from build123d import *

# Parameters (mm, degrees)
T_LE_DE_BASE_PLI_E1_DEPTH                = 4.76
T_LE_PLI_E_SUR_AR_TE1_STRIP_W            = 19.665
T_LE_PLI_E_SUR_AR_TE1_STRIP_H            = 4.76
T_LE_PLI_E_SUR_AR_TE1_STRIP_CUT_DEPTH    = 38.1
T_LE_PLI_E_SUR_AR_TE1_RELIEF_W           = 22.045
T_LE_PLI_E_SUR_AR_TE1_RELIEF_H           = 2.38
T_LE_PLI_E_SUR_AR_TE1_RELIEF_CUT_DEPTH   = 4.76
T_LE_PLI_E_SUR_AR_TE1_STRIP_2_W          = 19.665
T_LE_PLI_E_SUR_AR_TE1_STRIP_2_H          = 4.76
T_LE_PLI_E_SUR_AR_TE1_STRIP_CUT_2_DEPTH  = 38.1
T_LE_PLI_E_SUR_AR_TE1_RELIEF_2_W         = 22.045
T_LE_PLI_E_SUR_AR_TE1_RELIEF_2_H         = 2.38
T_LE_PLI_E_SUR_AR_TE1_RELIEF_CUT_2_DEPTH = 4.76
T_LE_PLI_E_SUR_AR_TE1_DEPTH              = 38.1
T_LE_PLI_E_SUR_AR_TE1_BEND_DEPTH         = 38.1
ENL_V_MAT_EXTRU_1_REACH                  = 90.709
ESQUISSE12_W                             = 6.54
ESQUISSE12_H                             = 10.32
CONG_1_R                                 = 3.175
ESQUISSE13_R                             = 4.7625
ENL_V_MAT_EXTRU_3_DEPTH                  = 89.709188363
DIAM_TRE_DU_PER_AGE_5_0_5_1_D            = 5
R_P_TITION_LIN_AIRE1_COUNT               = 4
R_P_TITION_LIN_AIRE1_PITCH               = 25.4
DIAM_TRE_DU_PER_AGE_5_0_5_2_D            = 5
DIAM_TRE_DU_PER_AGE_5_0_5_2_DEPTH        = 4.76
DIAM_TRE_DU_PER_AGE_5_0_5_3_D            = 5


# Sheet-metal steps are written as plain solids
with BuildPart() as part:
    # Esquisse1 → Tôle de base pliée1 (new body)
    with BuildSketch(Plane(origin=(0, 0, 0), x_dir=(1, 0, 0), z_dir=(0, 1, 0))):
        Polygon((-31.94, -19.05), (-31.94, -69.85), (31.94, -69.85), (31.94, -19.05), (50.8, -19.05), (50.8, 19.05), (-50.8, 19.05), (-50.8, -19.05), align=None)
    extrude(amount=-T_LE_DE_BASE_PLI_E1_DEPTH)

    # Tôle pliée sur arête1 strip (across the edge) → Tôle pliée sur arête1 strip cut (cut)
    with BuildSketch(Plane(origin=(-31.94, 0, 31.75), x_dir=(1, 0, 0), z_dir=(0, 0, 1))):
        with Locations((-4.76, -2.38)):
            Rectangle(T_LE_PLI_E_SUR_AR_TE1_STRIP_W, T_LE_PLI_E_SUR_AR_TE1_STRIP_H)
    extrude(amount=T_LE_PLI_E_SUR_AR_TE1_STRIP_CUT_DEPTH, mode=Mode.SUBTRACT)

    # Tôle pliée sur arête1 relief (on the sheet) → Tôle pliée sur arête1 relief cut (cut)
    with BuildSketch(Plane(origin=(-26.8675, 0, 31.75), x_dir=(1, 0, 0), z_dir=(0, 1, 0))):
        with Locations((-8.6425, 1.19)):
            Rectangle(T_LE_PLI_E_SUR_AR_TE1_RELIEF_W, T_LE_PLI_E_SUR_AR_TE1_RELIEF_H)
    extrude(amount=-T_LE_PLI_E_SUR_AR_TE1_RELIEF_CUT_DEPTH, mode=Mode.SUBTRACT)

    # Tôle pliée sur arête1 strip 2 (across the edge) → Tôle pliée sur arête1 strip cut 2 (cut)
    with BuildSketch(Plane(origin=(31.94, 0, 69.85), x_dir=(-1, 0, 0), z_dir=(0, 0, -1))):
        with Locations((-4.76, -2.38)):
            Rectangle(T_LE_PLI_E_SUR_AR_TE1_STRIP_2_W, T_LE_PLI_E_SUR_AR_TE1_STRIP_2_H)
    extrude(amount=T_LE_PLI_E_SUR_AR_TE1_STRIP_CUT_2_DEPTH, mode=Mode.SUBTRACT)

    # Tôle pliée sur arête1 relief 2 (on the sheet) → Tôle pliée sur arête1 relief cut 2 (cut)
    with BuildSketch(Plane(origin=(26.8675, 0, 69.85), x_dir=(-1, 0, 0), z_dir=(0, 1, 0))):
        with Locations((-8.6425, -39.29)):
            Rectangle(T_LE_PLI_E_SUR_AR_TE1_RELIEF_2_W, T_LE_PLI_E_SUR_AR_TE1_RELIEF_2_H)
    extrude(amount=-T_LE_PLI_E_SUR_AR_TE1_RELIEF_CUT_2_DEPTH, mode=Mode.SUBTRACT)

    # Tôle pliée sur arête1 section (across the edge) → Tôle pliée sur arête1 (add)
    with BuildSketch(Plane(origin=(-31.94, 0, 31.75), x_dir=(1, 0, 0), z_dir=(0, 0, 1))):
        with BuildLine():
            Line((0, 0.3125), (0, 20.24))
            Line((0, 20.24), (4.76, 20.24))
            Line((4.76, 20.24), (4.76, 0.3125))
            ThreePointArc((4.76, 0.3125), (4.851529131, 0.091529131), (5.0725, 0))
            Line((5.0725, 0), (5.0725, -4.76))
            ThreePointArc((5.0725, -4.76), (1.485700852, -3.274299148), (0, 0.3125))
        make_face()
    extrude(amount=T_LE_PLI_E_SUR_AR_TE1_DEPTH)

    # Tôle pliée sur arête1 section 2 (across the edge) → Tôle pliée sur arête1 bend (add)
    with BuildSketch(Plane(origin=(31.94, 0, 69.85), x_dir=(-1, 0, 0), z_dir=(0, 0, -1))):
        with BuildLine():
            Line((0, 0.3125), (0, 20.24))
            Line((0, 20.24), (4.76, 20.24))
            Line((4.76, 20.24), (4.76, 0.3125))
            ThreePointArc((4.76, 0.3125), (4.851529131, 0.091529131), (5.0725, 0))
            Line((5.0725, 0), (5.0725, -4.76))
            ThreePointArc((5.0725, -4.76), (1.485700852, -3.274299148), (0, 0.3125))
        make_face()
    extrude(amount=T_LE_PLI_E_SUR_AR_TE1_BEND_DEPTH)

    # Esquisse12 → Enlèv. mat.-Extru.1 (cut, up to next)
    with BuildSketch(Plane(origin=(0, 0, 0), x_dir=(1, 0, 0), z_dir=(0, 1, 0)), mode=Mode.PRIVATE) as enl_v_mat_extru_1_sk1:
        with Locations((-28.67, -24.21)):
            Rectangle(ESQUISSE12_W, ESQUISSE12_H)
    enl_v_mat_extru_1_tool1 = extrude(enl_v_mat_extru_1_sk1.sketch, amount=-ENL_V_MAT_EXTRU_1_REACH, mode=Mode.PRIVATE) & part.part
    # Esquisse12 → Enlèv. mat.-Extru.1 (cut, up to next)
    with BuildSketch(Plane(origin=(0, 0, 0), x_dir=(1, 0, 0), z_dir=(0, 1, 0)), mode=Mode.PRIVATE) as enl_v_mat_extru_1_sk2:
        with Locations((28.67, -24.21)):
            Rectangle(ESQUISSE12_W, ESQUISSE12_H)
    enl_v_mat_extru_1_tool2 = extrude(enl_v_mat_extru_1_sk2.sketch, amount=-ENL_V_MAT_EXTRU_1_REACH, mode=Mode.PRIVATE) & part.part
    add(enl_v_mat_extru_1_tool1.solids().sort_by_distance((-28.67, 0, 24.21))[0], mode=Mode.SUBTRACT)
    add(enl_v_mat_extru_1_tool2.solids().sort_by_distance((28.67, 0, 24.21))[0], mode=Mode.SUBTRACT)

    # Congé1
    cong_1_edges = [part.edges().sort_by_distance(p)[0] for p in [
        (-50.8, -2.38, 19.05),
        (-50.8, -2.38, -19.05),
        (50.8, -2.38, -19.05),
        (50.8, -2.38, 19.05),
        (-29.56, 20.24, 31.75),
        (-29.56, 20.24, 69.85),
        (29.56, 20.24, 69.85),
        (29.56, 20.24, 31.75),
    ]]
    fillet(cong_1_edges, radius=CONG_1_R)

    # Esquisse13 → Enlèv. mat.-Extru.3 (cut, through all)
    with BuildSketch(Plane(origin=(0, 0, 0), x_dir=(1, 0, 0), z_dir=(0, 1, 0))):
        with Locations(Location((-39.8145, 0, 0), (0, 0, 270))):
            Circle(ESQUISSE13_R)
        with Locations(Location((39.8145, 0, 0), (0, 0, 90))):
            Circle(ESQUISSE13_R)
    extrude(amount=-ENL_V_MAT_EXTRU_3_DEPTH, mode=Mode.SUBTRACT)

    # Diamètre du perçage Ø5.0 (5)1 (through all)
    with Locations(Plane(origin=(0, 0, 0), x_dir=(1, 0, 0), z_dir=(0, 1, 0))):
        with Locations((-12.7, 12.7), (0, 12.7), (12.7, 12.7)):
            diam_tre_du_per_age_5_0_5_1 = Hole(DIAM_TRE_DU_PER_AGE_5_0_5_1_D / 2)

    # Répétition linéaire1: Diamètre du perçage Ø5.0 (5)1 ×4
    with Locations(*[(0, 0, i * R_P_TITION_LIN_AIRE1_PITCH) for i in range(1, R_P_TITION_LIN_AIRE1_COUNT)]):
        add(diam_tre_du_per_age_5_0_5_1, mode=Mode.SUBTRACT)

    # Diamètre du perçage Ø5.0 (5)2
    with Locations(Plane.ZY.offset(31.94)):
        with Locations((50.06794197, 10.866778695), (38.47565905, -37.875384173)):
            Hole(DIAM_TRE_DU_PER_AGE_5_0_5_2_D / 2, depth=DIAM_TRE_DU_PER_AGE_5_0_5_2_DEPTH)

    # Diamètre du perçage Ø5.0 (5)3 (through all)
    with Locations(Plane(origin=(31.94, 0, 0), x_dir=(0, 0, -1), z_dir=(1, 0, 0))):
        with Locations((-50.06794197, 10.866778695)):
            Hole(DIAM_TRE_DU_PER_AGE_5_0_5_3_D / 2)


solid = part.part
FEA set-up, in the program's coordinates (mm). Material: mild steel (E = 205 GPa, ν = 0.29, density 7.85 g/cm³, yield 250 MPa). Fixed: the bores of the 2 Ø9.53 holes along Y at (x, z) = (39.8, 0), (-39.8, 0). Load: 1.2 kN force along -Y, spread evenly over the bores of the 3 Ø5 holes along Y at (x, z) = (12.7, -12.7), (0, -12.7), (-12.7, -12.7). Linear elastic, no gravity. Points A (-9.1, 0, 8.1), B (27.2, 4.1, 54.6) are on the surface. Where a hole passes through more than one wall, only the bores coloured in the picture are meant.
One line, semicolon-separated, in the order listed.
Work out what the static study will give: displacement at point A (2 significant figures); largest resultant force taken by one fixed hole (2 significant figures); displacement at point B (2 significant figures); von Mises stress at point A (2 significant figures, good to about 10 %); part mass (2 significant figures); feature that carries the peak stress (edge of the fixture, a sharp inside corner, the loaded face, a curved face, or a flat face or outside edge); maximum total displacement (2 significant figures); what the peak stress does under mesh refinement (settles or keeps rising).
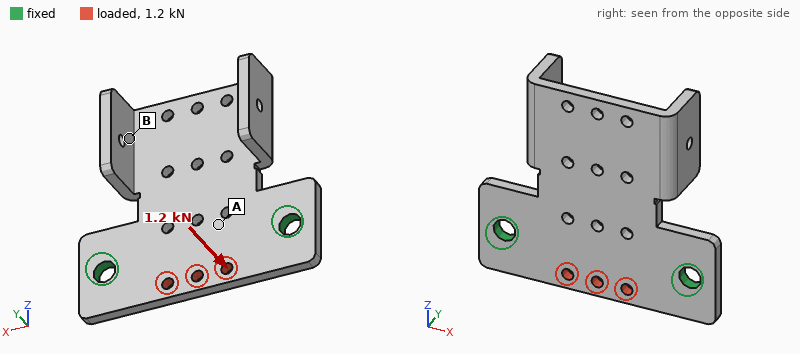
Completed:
16 µm; 600 N; 40 µm; 33 MPa; 300 g; edge of the fixture; 77 µm; keeps rising
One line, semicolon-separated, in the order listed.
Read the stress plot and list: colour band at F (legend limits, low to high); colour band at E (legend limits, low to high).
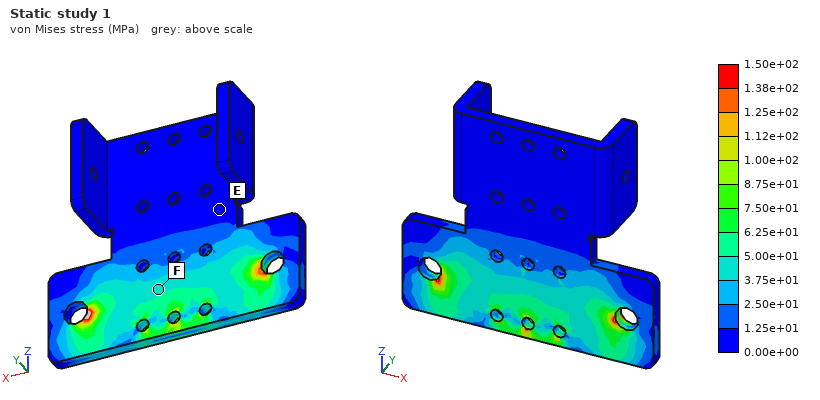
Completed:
3.75e+01 to 5.00e+01 MPa; 0.00e+00 to 1.25e+01 MPa
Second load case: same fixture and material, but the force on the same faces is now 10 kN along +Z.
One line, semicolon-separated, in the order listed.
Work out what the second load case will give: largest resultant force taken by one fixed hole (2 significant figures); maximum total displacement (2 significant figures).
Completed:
5.0 kN; 22 µm
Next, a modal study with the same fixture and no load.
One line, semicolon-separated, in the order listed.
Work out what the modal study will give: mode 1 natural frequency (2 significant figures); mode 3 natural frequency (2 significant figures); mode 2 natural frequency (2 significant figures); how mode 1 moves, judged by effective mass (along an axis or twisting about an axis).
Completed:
550 Hz; 2900 Hz; 1200 Hz; along Y
